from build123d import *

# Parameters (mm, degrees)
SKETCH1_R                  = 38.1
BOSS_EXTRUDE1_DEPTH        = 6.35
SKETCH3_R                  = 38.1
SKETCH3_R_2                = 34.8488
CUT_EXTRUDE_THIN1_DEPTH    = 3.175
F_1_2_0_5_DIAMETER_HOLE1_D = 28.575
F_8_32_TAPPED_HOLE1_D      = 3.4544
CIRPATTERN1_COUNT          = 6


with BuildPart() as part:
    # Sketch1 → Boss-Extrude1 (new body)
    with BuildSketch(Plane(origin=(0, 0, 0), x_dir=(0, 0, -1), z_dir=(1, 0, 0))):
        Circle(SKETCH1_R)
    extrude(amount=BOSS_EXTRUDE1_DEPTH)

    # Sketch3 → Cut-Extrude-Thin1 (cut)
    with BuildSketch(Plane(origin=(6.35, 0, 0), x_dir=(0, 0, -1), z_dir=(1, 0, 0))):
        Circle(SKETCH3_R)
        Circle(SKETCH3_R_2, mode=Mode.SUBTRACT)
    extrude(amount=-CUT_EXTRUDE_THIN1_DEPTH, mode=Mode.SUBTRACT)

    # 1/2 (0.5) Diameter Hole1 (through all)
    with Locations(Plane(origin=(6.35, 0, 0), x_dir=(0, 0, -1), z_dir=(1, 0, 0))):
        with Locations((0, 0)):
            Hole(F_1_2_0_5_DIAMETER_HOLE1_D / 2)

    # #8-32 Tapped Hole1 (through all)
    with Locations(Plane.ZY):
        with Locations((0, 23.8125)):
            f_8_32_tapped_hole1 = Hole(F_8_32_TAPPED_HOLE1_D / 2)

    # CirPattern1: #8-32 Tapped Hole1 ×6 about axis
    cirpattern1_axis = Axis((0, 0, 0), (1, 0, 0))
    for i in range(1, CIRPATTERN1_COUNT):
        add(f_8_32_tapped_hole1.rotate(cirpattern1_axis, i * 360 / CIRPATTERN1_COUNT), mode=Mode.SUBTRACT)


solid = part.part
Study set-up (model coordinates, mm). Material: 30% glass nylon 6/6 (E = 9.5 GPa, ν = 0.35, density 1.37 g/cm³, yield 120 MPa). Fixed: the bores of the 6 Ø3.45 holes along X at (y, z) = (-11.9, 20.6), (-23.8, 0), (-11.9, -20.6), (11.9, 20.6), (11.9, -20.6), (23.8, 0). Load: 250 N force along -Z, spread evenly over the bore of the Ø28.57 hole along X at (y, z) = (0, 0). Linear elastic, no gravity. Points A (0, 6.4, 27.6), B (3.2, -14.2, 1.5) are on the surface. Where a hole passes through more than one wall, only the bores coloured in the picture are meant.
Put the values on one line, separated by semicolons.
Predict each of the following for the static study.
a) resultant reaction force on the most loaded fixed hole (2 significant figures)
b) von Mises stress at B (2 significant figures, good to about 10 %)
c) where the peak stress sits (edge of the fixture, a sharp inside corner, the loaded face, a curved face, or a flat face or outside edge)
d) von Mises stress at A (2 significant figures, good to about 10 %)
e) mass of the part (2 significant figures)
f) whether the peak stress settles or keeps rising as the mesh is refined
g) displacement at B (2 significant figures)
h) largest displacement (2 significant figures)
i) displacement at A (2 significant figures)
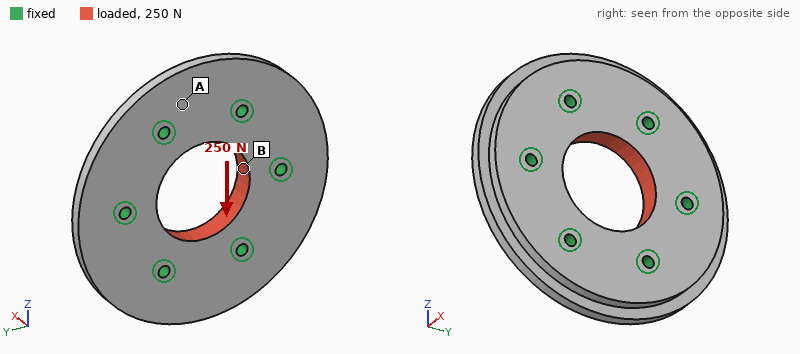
49 N; 0.76 MPa; edge of the fixture; 0.25 MPa; 30 g; keeps rising; 0.84 µm; 0.86 µm; 0.35 µm
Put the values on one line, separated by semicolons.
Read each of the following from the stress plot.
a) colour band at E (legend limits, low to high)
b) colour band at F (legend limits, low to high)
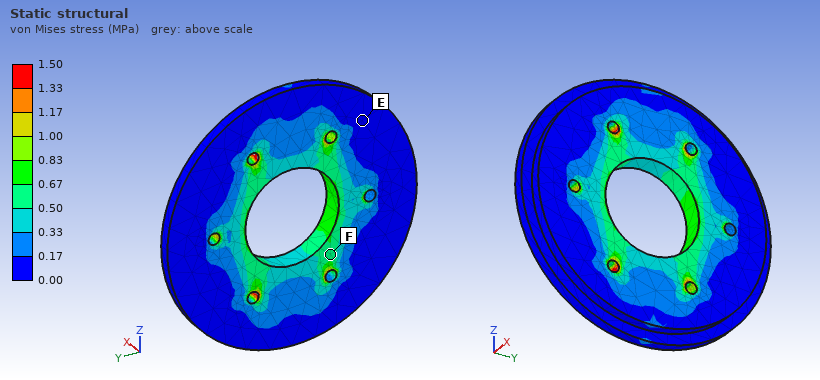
0.00 to 0.17 MPa; 0.50 to 0.67 MPa
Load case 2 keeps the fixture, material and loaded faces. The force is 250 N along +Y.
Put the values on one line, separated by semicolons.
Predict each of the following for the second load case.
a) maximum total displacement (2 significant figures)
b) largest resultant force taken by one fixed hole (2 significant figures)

0.85 µm; 54 N
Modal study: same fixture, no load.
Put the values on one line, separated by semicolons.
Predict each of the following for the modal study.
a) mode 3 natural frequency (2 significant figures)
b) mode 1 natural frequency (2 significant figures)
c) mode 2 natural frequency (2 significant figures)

9600 Hz; 9400 Hz; 9600 Hz
